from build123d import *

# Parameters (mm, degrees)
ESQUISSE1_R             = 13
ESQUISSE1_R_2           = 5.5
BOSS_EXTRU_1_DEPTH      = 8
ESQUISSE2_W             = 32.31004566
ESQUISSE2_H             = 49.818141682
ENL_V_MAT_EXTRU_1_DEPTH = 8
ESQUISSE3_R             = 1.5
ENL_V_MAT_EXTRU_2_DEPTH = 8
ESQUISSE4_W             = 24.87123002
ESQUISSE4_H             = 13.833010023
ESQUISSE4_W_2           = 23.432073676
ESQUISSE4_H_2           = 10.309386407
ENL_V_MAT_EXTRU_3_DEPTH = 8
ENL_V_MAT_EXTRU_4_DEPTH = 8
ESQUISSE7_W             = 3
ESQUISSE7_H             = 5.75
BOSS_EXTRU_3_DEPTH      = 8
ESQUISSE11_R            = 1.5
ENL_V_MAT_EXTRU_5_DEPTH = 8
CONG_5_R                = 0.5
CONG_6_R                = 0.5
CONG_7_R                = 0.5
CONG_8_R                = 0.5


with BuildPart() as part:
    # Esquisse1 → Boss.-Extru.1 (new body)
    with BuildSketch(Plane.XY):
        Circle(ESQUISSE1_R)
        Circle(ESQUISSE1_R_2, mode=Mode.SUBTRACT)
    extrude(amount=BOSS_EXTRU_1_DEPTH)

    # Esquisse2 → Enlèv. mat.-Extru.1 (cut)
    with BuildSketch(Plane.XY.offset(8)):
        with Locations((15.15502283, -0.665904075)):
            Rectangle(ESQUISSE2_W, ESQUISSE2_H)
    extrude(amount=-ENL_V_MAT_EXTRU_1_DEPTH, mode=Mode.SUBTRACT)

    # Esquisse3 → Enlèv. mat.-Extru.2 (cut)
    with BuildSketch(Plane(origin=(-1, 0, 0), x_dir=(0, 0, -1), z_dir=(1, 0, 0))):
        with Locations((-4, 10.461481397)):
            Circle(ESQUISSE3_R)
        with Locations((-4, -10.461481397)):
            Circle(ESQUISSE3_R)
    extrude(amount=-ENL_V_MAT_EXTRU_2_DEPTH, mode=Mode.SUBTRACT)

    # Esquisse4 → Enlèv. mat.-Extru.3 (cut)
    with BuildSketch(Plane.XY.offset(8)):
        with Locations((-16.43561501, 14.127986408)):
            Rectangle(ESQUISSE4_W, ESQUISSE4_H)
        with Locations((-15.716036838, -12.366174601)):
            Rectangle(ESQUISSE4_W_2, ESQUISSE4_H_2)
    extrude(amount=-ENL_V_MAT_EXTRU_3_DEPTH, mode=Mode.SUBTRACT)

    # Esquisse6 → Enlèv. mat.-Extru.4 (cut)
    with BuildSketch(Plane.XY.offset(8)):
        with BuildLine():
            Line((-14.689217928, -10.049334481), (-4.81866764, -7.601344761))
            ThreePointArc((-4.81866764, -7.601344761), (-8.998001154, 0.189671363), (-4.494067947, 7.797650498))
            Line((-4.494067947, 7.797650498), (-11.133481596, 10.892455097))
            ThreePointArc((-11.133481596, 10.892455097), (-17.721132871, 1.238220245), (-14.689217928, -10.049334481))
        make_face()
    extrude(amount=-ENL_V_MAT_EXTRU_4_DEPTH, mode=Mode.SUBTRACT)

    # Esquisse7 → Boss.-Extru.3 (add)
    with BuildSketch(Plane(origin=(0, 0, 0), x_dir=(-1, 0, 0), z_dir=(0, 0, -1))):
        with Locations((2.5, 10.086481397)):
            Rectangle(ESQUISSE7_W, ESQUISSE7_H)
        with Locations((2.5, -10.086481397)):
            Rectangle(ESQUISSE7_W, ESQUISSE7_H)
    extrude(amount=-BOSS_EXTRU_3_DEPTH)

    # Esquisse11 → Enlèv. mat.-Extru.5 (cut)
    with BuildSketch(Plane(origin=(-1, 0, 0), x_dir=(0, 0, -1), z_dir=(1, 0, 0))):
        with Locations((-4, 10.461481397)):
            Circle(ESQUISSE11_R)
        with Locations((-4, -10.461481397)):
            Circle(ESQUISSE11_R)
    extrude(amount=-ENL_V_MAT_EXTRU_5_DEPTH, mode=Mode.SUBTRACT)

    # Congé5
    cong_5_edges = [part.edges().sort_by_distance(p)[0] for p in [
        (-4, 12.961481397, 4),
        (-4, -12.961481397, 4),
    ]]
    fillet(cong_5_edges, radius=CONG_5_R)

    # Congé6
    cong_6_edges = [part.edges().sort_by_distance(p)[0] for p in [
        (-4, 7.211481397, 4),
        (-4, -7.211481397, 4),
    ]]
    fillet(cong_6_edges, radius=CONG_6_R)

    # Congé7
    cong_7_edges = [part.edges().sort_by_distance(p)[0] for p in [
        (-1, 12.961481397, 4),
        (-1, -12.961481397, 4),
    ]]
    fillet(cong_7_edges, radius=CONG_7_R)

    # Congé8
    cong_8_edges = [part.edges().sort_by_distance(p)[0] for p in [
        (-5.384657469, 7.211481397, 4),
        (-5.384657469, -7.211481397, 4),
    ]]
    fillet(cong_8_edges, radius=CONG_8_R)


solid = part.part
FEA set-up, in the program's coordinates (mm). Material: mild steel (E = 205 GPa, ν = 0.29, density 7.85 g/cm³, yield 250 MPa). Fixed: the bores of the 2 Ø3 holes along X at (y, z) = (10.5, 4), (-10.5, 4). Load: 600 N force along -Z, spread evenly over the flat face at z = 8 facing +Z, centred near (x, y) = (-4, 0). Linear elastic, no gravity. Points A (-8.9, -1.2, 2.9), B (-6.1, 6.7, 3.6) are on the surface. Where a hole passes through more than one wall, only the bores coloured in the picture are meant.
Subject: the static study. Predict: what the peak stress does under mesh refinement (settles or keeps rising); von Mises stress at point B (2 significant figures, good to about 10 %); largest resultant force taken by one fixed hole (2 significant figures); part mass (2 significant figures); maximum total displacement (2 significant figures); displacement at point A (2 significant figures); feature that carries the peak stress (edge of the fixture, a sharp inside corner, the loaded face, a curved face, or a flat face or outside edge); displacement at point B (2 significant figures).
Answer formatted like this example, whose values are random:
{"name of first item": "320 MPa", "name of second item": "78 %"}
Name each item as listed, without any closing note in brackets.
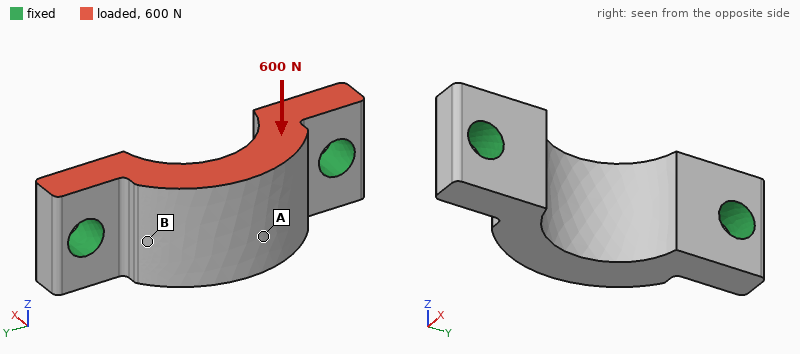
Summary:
{"what the peak stress does under mesh refinement": "keeps rising", "von Mises stress at point B": "23 MPa", "largest resultant force taken by one fixed hole": "300 N", "part mass": "5.8 g", "maximum total displacement": "4.7 µm", "displacement at point A": "4.1 µm", "feature that carries the peak stress": "edge of the fixture", "displacement at point B": "2.2 µm"}
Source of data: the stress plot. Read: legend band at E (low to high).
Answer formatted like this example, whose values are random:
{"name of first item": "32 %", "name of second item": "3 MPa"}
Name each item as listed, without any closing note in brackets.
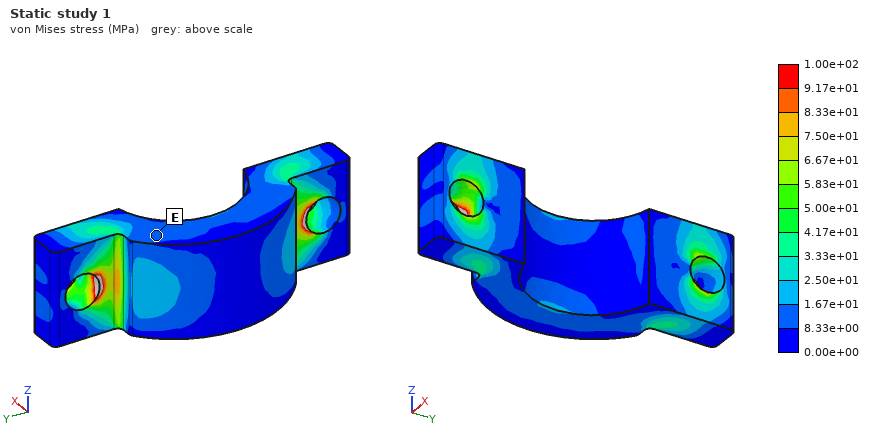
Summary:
{"legend band at E": "8.33e+00 to 1.67e+01 MPa"}
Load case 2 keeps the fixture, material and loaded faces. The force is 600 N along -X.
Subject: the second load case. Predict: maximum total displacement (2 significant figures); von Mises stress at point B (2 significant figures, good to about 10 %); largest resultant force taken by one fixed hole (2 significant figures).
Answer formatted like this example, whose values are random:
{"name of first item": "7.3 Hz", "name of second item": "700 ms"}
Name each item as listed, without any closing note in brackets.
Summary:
{"maximum total displacement": "6.0 µm", "von Mises stress at point B": "20 MPa", "largest resultant force taken by one fixed hole": "330 N"}
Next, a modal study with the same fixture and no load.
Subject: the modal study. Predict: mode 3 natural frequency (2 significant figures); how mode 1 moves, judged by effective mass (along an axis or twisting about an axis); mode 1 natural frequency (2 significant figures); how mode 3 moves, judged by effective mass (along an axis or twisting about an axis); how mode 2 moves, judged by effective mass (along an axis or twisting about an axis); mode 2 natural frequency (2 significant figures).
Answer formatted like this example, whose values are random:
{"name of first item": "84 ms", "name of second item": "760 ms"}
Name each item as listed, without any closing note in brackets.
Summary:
{"mode 3 natural frequency": "67 kHz", "how mode 1 moves, judged by effective mass": "along Z", "mode 1 natural frequency": "28 kHz", "how mode 3 moves, judged by effective mass": "along Y", "how mode 2 moves, judged by effective mass": "along X", "mode 2 natural frequency": "51 kHz"}
